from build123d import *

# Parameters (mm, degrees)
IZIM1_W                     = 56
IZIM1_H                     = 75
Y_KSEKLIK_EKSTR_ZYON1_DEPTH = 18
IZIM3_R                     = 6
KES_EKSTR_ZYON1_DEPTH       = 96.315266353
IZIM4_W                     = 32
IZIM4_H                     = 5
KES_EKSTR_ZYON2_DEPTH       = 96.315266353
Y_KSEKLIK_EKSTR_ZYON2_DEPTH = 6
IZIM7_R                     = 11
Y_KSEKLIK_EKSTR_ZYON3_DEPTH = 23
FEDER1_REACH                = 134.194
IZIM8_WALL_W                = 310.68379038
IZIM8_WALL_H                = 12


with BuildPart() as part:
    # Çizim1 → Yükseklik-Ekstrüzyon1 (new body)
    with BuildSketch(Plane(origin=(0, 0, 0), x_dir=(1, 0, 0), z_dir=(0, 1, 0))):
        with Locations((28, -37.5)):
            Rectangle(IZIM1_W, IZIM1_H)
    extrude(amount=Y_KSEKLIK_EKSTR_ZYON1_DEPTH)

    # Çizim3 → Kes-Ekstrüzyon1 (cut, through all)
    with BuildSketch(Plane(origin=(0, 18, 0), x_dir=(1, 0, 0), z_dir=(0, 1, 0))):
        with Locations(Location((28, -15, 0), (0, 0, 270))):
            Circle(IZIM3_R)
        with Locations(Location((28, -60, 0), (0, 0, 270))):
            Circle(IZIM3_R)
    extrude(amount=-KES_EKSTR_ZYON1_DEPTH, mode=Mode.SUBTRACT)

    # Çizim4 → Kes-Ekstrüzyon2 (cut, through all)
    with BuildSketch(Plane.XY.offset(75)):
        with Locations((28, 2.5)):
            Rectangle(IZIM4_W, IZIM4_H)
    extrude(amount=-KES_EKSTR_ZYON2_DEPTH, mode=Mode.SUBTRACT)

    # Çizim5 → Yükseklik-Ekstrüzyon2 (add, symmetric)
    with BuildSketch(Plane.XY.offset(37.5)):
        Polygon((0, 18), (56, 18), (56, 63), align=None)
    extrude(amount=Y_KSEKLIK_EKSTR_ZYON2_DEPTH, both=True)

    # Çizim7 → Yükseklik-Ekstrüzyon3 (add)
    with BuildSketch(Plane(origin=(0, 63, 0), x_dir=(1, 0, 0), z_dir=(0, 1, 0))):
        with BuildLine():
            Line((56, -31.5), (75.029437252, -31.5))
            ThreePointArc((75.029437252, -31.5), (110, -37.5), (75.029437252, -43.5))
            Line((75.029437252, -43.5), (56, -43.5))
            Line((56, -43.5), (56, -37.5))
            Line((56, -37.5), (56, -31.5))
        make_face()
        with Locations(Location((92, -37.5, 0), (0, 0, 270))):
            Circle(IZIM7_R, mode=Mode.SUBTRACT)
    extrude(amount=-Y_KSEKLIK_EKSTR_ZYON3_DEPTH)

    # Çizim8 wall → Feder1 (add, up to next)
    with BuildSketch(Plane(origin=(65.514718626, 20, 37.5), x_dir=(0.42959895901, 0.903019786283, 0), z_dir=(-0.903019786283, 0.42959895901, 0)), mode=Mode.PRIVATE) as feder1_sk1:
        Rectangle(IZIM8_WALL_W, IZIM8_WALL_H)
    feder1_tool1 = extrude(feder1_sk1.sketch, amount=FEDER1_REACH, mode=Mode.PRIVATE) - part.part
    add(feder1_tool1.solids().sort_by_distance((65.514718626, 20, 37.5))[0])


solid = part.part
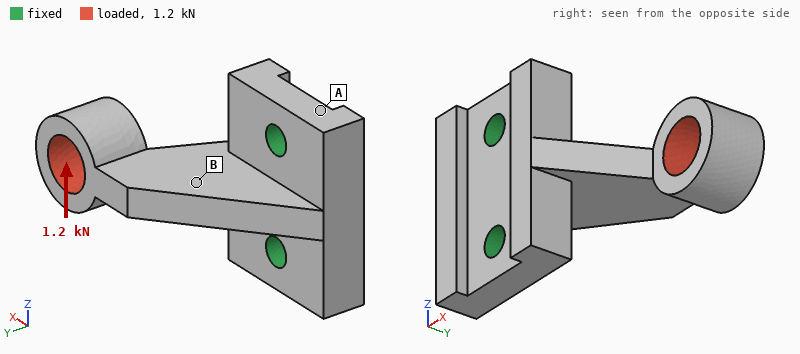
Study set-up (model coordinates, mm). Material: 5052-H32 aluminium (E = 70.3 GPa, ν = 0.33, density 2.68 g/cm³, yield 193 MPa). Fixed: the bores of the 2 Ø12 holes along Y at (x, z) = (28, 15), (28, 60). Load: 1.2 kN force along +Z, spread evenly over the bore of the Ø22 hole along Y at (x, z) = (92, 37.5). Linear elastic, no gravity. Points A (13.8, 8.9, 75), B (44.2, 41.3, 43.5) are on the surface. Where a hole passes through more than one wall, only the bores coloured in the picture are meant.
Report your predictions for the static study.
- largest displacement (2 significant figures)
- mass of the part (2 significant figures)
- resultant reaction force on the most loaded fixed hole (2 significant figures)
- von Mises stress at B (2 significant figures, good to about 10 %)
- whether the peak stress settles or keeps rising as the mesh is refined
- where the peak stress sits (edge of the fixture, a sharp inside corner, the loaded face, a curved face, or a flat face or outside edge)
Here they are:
0.42 mm
270 g
2.0 kN
45 MPa
keeps rising
a sharp inside corner
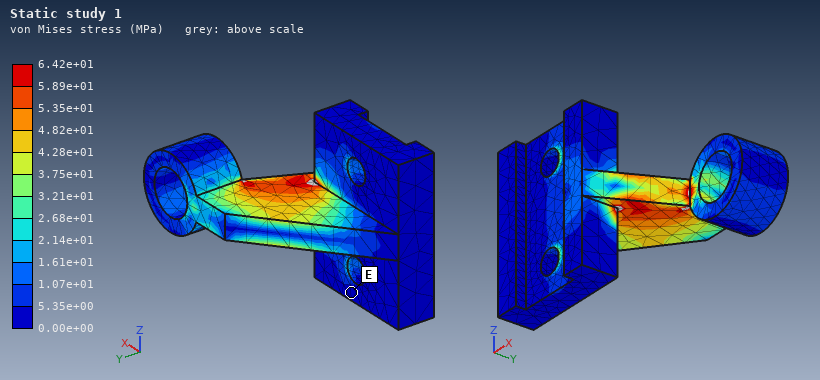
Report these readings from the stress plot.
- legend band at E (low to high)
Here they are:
0.00e+00 to 5.35e+00 MPa
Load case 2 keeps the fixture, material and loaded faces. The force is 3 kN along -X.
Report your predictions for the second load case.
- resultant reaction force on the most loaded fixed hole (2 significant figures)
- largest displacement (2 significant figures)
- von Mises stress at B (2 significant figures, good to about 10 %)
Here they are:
1.5 kN
0.14 mm
15 MPa
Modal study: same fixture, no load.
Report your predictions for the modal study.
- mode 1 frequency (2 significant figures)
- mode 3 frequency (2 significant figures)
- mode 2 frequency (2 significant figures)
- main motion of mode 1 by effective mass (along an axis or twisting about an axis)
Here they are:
1500 Hz
4100 Hz
2500 Hz
along Z
